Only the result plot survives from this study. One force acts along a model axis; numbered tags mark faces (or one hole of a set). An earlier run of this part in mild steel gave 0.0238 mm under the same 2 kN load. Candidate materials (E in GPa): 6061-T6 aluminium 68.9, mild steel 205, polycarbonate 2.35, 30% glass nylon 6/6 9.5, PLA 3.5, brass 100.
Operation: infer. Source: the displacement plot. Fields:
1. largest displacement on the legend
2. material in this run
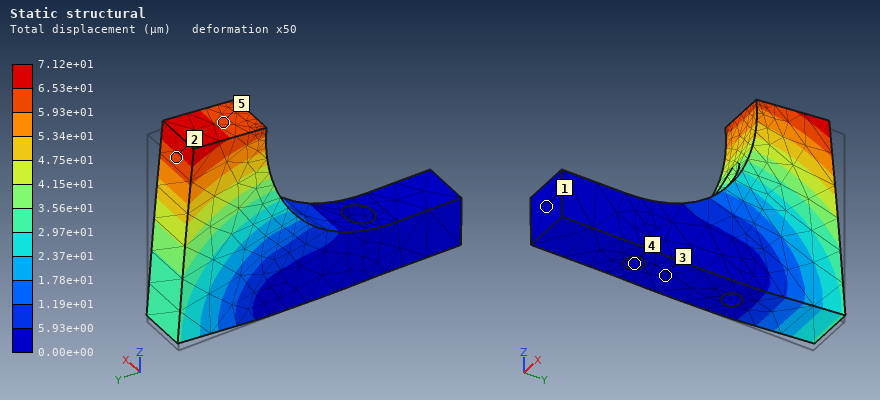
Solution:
7.12e+01 µm
6061-T6 aluminium
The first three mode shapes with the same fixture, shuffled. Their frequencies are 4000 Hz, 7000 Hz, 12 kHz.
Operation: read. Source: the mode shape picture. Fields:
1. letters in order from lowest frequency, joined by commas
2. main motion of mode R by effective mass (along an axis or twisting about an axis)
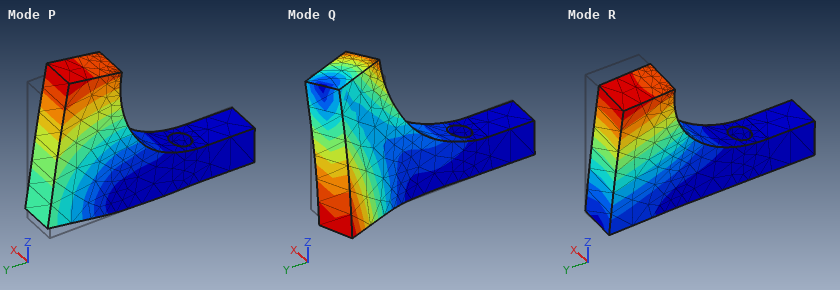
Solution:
R, P, Q
along X
